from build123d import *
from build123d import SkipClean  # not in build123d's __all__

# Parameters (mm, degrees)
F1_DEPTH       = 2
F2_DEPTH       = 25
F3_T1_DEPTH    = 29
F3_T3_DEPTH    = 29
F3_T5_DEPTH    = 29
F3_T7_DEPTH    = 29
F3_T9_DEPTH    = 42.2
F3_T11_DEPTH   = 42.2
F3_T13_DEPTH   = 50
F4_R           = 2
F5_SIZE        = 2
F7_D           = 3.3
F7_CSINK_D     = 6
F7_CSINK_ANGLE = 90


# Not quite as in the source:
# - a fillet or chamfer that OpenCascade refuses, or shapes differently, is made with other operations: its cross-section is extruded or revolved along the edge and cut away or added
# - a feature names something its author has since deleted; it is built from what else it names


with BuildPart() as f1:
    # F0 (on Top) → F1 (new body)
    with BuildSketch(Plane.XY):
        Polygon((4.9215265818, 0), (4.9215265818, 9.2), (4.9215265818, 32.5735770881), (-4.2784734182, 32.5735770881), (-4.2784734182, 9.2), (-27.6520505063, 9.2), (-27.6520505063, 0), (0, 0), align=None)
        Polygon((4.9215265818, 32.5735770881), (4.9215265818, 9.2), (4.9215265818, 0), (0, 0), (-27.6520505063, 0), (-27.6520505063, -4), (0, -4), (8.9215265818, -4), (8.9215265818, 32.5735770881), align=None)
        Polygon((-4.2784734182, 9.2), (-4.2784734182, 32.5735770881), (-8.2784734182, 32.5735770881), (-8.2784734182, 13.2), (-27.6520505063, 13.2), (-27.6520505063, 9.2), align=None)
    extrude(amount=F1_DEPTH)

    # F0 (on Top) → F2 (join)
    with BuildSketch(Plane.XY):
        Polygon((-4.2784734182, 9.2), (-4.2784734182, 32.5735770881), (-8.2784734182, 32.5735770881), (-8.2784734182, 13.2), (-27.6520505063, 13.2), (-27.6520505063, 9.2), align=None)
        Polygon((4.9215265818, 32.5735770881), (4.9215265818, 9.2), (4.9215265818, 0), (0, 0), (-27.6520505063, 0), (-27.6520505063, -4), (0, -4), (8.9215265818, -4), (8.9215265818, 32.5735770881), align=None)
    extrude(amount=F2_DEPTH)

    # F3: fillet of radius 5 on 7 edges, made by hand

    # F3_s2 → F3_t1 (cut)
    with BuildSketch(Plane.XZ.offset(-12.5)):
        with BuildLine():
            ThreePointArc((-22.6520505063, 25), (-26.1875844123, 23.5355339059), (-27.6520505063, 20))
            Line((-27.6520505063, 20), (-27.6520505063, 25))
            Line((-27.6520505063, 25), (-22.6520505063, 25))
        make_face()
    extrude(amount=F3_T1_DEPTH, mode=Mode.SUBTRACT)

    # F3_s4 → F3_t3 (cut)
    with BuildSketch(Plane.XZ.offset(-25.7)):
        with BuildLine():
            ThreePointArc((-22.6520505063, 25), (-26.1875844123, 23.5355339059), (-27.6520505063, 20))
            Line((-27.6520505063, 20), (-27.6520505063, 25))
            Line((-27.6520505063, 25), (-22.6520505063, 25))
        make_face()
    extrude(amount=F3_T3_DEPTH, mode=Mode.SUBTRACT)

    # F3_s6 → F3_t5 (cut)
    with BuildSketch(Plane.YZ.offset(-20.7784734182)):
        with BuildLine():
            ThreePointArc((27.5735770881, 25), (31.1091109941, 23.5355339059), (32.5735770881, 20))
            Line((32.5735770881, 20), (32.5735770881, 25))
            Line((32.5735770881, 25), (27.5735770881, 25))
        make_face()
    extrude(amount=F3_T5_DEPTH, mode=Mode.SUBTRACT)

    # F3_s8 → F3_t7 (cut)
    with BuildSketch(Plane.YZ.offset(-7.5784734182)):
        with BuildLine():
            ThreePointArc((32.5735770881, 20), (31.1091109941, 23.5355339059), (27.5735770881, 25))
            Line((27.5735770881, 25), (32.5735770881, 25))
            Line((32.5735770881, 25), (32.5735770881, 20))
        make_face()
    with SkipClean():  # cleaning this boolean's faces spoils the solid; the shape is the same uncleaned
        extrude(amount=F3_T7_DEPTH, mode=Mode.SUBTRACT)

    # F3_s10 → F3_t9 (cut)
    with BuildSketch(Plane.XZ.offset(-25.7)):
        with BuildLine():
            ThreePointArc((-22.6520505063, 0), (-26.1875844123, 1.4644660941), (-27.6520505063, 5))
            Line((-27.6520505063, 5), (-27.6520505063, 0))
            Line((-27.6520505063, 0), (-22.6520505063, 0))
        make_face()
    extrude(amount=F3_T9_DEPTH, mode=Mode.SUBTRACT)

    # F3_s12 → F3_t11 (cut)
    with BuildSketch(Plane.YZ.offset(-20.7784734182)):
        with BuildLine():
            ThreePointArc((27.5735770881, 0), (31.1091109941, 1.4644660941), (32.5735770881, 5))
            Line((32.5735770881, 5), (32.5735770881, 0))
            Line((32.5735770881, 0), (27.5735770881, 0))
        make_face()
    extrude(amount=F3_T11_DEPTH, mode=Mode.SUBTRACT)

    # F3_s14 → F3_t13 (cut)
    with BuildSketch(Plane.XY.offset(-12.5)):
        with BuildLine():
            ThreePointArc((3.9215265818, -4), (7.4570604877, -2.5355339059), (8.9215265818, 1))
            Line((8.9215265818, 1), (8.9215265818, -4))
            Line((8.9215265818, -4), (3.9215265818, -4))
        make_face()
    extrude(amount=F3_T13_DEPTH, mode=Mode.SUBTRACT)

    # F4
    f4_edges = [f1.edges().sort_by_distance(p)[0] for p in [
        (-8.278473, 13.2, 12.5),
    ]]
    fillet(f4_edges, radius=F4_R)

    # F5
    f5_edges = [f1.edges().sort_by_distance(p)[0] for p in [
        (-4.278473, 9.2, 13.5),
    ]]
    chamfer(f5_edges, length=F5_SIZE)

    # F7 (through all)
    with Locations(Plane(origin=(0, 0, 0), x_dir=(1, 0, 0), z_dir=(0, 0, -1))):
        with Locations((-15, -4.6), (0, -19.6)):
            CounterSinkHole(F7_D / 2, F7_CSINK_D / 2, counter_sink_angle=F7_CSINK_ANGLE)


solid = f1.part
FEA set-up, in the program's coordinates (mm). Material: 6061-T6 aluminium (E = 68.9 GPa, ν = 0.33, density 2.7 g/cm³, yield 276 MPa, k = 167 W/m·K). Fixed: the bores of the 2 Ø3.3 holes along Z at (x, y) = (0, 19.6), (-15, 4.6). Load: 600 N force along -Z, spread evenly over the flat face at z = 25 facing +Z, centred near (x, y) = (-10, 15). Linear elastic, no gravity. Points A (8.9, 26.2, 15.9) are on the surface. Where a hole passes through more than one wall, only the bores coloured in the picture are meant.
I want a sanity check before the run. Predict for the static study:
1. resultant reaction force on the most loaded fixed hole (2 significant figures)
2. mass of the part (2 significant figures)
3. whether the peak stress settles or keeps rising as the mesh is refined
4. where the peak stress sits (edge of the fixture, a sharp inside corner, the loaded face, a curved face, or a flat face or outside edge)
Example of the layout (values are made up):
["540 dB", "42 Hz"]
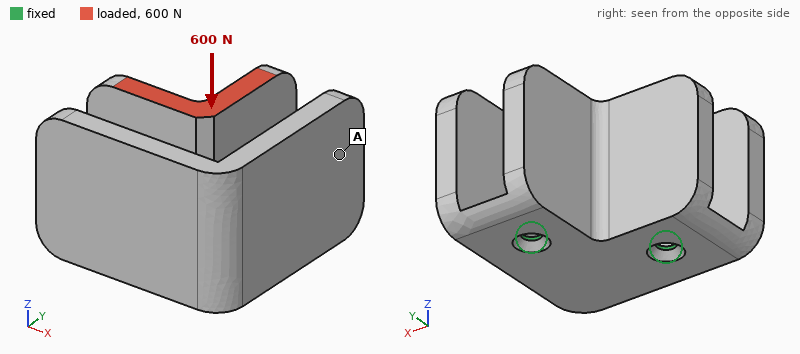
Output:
["310 N", "32 g", "keeps rising", "edge of the fixture"]
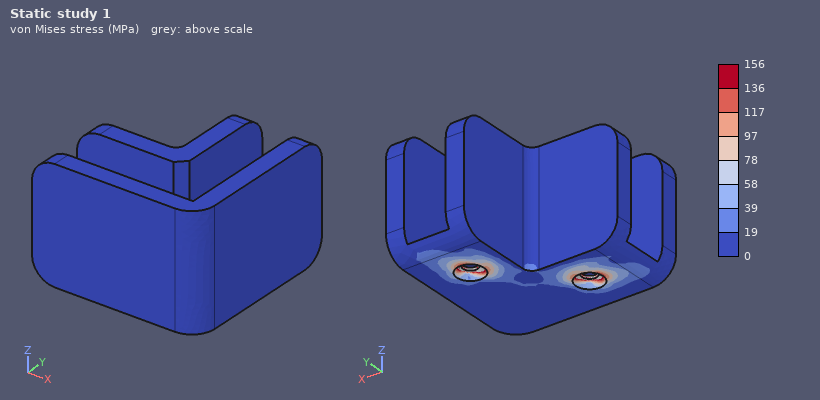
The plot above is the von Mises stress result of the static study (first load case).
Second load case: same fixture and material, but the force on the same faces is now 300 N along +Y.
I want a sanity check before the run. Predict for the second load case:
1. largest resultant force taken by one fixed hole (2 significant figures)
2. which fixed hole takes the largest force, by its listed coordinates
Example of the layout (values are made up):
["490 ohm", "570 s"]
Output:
["380 N", "(0, 19.6)"]
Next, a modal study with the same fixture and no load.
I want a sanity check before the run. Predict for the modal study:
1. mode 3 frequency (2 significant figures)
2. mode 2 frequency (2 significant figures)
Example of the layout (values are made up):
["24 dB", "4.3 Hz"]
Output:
["2900 Hz", "2800 Hz"]
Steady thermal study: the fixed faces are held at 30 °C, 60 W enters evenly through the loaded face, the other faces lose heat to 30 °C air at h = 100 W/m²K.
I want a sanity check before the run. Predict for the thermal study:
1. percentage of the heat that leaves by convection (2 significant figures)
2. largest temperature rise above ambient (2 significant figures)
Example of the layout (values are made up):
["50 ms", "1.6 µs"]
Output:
["30 %", "82 K"]
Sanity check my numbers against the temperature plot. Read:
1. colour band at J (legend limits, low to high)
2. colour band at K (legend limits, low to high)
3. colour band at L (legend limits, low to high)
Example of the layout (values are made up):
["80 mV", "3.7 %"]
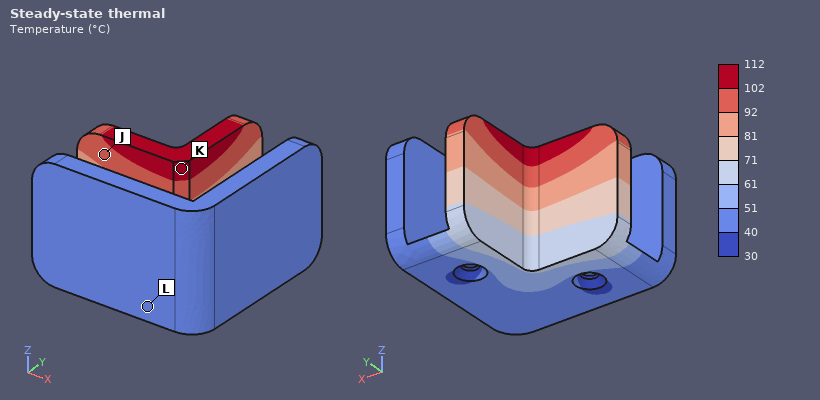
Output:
["92 to 102 °C", "102 to 112 °C", "40 to 51 °C"]
